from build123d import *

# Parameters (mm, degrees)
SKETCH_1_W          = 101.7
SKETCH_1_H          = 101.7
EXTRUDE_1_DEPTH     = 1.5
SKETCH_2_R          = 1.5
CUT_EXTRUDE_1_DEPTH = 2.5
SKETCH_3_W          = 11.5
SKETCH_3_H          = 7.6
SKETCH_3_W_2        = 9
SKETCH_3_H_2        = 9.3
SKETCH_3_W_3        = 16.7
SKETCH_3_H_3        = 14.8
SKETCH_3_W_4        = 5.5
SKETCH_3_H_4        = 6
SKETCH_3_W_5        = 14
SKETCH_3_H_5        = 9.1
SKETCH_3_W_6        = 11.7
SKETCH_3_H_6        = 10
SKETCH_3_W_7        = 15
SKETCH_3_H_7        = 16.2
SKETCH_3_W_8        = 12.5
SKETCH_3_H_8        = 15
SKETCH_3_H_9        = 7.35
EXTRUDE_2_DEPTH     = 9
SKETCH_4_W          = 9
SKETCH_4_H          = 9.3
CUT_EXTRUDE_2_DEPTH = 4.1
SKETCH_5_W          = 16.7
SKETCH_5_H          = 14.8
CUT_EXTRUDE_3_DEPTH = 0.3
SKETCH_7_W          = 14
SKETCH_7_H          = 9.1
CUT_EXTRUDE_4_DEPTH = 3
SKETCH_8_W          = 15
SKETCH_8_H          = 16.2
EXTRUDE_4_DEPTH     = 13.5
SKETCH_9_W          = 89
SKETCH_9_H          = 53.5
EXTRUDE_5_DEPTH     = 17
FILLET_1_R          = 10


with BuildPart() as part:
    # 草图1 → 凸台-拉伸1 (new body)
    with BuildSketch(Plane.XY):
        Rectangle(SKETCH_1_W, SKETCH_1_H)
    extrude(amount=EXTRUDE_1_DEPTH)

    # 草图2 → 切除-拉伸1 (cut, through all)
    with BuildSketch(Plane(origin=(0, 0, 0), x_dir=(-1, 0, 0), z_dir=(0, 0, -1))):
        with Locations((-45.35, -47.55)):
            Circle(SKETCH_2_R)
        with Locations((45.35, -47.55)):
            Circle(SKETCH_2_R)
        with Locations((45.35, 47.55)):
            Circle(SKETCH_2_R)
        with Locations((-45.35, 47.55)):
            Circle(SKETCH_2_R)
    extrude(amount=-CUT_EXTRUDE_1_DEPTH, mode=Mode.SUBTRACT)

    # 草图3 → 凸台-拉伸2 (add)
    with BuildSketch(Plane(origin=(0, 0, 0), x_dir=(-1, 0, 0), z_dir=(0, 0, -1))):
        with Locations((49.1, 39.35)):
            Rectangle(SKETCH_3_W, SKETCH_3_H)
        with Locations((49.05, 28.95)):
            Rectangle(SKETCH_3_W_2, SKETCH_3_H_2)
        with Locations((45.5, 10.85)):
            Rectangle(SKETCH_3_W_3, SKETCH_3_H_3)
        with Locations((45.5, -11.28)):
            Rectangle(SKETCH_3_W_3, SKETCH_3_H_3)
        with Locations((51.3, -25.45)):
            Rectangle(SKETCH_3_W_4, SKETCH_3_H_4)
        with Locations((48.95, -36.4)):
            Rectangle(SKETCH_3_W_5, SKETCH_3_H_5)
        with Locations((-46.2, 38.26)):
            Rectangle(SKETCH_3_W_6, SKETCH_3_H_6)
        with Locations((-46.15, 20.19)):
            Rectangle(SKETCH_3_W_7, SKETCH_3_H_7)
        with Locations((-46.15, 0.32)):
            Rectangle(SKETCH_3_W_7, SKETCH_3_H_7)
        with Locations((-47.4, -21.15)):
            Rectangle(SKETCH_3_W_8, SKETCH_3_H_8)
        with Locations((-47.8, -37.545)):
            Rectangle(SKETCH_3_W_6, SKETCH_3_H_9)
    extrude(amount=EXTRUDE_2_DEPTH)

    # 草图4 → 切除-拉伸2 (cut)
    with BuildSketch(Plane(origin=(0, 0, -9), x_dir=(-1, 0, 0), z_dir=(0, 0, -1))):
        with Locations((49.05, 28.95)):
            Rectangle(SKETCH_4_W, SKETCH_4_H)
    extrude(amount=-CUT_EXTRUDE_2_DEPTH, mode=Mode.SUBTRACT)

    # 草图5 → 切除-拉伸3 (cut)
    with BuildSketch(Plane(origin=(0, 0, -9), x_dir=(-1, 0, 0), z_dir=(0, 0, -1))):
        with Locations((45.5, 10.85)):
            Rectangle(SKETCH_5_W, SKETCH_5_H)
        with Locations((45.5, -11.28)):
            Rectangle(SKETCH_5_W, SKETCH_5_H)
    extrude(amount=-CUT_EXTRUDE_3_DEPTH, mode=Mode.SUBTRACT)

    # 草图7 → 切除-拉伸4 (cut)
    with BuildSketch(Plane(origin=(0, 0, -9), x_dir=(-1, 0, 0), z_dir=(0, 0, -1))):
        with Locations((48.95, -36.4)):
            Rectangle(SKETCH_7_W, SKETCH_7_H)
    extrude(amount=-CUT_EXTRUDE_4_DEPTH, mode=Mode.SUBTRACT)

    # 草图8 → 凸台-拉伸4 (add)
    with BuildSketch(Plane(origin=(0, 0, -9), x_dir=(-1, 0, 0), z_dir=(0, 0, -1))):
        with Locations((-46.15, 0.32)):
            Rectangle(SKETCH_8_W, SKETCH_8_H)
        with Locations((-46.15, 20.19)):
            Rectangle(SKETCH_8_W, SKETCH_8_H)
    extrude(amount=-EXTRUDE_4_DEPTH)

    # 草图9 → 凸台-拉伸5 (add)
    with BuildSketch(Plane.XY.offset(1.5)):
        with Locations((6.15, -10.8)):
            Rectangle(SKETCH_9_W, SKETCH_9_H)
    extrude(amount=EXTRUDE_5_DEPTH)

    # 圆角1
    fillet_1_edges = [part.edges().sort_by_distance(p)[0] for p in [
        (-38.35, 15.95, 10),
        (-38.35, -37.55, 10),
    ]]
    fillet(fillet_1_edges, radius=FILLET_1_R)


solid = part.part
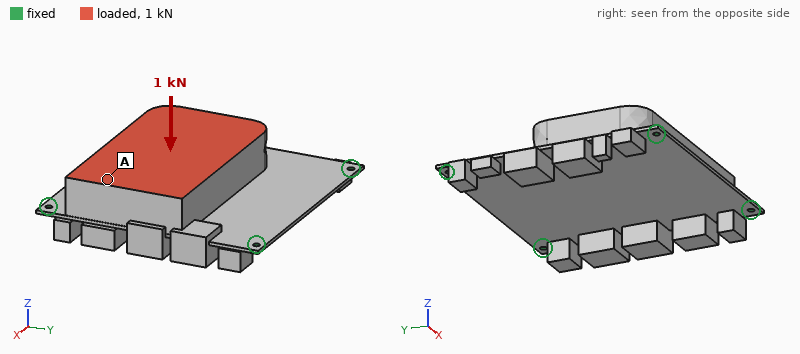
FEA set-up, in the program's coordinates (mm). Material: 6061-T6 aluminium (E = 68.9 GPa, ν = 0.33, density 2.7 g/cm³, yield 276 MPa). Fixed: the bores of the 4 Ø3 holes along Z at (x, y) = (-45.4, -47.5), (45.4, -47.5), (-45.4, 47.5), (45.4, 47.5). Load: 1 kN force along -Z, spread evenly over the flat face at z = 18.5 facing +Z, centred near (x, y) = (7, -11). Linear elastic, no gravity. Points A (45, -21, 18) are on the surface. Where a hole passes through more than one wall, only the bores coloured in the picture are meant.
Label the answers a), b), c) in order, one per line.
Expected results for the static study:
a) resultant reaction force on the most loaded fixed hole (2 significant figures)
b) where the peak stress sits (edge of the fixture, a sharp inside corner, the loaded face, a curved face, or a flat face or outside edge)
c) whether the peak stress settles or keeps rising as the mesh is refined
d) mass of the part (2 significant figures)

a) 340 N
b) edge of the fixture
c) keeps rising
d) 300 g
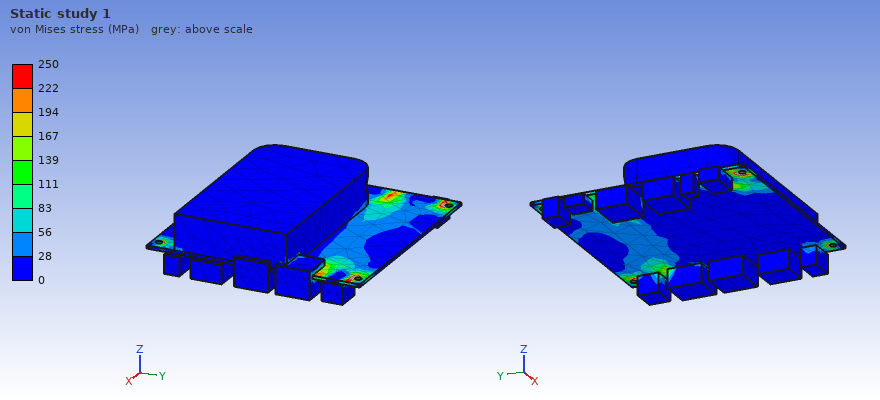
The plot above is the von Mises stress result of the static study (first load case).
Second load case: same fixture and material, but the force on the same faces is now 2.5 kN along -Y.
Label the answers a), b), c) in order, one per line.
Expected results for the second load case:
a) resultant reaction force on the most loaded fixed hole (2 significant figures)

a) 870 N
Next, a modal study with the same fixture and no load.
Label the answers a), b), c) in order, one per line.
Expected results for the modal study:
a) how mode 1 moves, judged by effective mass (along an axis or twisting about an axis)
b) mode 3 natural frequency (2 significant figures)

a) along Z
b) 1700 Hz
